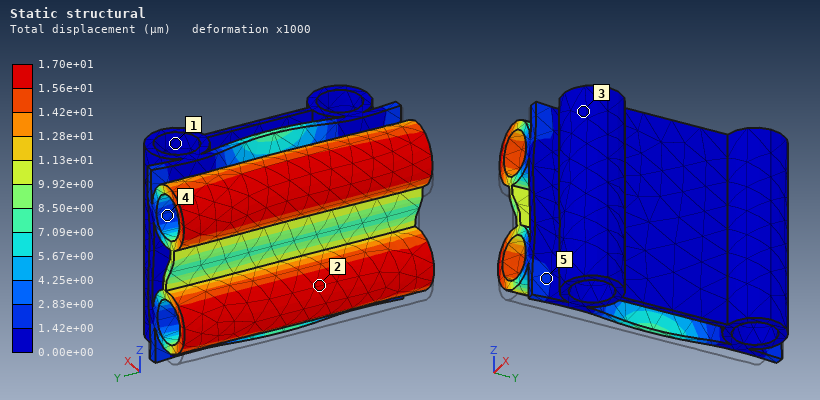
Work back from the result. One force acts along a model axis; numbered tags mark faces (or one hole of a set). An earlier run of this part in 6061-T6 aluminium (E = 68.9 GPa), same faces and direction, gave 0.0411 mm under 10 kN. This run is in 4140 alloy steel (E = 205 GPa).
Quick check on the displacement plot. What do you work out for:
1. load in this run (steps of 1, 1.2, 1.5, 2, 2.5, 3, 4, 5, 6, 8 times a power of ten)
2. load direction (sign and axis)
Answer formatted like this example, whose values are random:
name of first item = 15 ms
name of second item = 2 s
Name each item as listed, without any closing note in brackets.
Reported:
load in this run = 12 kN
load direction = +Z
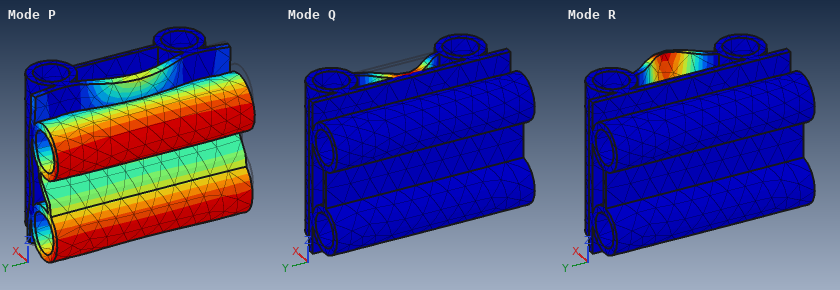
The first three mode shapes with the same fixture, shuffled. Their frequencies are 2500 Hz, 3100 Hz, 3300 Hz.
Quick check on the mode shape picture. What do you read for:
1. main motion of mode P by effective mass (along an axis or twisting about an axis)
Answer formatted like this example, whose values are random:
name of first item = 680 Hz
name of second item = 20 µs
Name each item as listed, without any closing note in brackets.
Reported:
main motion of mode P by effective mass = along Z
